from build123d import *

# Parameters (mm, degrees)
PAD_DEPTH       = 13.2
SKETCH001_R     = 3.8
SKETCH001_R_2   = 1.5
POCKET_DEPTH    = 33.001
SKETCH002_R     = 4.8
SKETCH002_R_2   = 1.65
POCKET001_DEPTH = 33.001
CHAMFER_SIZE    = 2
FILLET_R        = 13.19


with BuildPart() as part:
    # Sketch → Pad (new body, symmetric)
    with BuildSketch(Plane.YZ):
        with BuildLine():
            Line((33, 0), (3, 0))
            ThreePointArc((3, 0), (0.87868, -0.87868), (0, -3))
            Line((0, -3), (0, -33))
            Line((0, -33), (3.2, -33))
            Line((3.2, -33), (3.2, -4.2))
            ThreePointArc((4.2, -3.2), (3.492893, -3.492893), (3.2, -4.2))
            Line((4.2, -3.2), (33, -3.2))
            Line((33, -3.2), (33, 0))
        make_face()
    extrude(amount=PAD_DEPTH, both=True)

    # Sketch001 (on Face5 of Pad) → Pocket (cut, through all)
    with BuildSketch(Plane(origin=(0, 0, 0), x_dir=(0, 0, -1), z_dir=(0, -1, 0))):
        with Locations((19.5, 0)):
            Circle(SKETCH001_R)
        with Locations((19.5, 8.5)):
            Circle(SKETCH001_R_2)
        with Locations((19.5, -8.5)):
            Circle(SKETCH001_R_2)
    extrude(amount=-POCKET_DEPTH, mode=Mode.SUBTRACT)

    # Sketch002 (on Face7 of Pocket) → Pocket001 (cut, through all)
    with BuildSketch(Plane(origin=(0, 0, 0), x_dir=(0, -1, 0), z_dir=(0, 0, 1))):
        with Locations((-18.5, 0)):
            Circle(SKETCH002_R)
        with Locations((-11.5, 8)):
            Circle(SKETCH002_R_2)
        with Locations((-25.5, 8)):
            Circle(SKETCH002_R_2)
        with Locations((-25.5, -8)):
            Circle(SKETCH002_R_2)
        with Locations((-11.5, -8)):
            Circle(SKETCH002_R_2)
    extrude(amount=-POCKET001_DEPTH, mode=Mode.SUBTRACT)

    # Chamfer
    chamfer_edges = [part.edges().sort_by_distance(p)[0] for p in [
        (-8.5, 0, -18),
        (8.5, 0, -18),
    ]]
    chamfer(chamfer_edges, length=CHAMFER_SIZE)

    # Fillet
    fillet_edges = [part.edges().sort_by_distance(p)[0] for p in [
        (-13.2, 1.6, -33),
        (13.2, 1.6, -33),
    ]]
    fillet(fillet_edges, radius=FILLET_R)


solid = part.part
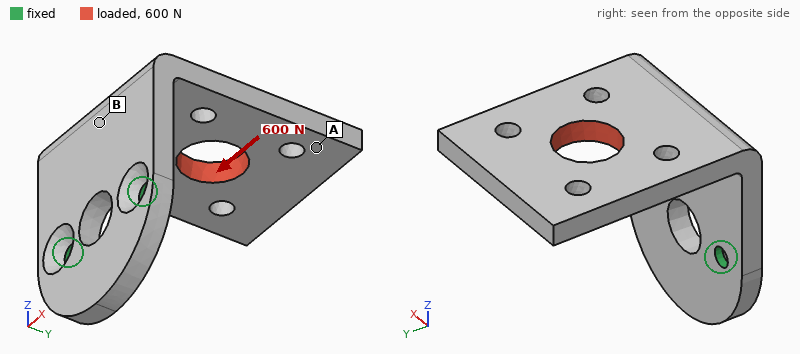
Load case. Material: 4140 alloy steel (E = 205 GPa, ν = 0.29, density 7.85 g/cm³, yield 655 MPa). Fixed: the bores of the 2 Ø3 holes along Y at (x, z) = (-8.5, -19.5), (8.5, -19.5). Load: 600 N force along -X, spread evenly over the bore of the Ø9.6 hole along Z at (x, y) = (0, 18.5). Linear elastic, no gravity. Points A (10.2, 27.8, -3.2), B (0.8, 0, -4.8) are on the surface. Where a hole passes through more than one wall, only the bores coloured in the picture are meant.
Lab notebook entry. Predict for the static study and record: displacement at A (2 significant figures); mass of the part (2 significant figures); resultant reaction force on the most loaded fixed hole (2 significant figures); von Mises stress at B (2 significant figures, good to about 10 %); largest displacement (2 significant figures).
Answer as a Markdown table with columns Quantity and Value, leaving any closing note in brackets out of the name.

| Quantity | Value |
|---|---|
| displacement at A | 0.17 mm |
| mass of the part | 35 g |
| resultant reaction force on the most loaded fixed hole | 790 N |
| von Mises stress at B | 120 MPa |
| largest displacement | 0.21 mm |
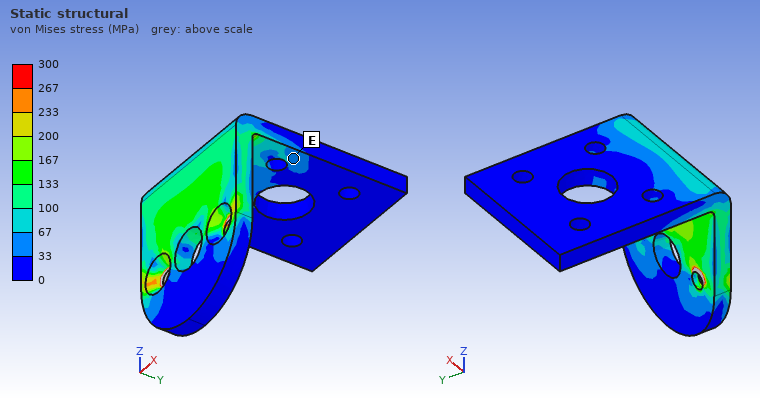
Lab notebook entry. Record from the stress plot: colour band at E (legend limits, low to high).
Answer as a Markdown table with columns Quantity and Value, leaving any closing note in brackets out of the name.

| Quantity | Value |
|---|---|
| colour band at E | 33 to 67 MPa |
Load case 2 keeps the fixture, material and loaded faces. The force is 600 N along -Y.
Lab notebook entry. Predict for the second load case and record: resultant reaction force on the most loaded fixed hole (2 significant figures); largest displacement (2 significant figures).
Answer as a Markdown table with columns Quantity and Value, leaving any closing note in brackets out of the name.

| Quantity | Value |
|---|---|
| resultant reaction force on the most loaded fixed hole | 320 N |
| largest displacement | 0.41 mm |
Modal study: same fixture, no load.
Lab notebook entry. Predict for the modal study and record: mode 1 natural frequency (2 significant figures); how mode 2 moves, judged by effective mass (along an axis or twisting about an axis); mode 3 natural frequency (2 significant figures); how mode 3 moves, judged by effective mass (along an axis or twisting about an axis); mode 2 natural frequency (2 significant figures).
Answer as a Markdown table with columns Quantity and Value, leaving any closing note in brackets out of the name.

| Quantity | Value |
|---|---|
| mode 1 natural frequency | 1200 Hz |
| how mode 2 moves, judged by effective mass | along X |
| mode 3 natural frequency | 3600 Hz |
| how mode 3 moves, judged by effective mass | along Y |
| mode 2 natural frequency | 2400 Hz |
